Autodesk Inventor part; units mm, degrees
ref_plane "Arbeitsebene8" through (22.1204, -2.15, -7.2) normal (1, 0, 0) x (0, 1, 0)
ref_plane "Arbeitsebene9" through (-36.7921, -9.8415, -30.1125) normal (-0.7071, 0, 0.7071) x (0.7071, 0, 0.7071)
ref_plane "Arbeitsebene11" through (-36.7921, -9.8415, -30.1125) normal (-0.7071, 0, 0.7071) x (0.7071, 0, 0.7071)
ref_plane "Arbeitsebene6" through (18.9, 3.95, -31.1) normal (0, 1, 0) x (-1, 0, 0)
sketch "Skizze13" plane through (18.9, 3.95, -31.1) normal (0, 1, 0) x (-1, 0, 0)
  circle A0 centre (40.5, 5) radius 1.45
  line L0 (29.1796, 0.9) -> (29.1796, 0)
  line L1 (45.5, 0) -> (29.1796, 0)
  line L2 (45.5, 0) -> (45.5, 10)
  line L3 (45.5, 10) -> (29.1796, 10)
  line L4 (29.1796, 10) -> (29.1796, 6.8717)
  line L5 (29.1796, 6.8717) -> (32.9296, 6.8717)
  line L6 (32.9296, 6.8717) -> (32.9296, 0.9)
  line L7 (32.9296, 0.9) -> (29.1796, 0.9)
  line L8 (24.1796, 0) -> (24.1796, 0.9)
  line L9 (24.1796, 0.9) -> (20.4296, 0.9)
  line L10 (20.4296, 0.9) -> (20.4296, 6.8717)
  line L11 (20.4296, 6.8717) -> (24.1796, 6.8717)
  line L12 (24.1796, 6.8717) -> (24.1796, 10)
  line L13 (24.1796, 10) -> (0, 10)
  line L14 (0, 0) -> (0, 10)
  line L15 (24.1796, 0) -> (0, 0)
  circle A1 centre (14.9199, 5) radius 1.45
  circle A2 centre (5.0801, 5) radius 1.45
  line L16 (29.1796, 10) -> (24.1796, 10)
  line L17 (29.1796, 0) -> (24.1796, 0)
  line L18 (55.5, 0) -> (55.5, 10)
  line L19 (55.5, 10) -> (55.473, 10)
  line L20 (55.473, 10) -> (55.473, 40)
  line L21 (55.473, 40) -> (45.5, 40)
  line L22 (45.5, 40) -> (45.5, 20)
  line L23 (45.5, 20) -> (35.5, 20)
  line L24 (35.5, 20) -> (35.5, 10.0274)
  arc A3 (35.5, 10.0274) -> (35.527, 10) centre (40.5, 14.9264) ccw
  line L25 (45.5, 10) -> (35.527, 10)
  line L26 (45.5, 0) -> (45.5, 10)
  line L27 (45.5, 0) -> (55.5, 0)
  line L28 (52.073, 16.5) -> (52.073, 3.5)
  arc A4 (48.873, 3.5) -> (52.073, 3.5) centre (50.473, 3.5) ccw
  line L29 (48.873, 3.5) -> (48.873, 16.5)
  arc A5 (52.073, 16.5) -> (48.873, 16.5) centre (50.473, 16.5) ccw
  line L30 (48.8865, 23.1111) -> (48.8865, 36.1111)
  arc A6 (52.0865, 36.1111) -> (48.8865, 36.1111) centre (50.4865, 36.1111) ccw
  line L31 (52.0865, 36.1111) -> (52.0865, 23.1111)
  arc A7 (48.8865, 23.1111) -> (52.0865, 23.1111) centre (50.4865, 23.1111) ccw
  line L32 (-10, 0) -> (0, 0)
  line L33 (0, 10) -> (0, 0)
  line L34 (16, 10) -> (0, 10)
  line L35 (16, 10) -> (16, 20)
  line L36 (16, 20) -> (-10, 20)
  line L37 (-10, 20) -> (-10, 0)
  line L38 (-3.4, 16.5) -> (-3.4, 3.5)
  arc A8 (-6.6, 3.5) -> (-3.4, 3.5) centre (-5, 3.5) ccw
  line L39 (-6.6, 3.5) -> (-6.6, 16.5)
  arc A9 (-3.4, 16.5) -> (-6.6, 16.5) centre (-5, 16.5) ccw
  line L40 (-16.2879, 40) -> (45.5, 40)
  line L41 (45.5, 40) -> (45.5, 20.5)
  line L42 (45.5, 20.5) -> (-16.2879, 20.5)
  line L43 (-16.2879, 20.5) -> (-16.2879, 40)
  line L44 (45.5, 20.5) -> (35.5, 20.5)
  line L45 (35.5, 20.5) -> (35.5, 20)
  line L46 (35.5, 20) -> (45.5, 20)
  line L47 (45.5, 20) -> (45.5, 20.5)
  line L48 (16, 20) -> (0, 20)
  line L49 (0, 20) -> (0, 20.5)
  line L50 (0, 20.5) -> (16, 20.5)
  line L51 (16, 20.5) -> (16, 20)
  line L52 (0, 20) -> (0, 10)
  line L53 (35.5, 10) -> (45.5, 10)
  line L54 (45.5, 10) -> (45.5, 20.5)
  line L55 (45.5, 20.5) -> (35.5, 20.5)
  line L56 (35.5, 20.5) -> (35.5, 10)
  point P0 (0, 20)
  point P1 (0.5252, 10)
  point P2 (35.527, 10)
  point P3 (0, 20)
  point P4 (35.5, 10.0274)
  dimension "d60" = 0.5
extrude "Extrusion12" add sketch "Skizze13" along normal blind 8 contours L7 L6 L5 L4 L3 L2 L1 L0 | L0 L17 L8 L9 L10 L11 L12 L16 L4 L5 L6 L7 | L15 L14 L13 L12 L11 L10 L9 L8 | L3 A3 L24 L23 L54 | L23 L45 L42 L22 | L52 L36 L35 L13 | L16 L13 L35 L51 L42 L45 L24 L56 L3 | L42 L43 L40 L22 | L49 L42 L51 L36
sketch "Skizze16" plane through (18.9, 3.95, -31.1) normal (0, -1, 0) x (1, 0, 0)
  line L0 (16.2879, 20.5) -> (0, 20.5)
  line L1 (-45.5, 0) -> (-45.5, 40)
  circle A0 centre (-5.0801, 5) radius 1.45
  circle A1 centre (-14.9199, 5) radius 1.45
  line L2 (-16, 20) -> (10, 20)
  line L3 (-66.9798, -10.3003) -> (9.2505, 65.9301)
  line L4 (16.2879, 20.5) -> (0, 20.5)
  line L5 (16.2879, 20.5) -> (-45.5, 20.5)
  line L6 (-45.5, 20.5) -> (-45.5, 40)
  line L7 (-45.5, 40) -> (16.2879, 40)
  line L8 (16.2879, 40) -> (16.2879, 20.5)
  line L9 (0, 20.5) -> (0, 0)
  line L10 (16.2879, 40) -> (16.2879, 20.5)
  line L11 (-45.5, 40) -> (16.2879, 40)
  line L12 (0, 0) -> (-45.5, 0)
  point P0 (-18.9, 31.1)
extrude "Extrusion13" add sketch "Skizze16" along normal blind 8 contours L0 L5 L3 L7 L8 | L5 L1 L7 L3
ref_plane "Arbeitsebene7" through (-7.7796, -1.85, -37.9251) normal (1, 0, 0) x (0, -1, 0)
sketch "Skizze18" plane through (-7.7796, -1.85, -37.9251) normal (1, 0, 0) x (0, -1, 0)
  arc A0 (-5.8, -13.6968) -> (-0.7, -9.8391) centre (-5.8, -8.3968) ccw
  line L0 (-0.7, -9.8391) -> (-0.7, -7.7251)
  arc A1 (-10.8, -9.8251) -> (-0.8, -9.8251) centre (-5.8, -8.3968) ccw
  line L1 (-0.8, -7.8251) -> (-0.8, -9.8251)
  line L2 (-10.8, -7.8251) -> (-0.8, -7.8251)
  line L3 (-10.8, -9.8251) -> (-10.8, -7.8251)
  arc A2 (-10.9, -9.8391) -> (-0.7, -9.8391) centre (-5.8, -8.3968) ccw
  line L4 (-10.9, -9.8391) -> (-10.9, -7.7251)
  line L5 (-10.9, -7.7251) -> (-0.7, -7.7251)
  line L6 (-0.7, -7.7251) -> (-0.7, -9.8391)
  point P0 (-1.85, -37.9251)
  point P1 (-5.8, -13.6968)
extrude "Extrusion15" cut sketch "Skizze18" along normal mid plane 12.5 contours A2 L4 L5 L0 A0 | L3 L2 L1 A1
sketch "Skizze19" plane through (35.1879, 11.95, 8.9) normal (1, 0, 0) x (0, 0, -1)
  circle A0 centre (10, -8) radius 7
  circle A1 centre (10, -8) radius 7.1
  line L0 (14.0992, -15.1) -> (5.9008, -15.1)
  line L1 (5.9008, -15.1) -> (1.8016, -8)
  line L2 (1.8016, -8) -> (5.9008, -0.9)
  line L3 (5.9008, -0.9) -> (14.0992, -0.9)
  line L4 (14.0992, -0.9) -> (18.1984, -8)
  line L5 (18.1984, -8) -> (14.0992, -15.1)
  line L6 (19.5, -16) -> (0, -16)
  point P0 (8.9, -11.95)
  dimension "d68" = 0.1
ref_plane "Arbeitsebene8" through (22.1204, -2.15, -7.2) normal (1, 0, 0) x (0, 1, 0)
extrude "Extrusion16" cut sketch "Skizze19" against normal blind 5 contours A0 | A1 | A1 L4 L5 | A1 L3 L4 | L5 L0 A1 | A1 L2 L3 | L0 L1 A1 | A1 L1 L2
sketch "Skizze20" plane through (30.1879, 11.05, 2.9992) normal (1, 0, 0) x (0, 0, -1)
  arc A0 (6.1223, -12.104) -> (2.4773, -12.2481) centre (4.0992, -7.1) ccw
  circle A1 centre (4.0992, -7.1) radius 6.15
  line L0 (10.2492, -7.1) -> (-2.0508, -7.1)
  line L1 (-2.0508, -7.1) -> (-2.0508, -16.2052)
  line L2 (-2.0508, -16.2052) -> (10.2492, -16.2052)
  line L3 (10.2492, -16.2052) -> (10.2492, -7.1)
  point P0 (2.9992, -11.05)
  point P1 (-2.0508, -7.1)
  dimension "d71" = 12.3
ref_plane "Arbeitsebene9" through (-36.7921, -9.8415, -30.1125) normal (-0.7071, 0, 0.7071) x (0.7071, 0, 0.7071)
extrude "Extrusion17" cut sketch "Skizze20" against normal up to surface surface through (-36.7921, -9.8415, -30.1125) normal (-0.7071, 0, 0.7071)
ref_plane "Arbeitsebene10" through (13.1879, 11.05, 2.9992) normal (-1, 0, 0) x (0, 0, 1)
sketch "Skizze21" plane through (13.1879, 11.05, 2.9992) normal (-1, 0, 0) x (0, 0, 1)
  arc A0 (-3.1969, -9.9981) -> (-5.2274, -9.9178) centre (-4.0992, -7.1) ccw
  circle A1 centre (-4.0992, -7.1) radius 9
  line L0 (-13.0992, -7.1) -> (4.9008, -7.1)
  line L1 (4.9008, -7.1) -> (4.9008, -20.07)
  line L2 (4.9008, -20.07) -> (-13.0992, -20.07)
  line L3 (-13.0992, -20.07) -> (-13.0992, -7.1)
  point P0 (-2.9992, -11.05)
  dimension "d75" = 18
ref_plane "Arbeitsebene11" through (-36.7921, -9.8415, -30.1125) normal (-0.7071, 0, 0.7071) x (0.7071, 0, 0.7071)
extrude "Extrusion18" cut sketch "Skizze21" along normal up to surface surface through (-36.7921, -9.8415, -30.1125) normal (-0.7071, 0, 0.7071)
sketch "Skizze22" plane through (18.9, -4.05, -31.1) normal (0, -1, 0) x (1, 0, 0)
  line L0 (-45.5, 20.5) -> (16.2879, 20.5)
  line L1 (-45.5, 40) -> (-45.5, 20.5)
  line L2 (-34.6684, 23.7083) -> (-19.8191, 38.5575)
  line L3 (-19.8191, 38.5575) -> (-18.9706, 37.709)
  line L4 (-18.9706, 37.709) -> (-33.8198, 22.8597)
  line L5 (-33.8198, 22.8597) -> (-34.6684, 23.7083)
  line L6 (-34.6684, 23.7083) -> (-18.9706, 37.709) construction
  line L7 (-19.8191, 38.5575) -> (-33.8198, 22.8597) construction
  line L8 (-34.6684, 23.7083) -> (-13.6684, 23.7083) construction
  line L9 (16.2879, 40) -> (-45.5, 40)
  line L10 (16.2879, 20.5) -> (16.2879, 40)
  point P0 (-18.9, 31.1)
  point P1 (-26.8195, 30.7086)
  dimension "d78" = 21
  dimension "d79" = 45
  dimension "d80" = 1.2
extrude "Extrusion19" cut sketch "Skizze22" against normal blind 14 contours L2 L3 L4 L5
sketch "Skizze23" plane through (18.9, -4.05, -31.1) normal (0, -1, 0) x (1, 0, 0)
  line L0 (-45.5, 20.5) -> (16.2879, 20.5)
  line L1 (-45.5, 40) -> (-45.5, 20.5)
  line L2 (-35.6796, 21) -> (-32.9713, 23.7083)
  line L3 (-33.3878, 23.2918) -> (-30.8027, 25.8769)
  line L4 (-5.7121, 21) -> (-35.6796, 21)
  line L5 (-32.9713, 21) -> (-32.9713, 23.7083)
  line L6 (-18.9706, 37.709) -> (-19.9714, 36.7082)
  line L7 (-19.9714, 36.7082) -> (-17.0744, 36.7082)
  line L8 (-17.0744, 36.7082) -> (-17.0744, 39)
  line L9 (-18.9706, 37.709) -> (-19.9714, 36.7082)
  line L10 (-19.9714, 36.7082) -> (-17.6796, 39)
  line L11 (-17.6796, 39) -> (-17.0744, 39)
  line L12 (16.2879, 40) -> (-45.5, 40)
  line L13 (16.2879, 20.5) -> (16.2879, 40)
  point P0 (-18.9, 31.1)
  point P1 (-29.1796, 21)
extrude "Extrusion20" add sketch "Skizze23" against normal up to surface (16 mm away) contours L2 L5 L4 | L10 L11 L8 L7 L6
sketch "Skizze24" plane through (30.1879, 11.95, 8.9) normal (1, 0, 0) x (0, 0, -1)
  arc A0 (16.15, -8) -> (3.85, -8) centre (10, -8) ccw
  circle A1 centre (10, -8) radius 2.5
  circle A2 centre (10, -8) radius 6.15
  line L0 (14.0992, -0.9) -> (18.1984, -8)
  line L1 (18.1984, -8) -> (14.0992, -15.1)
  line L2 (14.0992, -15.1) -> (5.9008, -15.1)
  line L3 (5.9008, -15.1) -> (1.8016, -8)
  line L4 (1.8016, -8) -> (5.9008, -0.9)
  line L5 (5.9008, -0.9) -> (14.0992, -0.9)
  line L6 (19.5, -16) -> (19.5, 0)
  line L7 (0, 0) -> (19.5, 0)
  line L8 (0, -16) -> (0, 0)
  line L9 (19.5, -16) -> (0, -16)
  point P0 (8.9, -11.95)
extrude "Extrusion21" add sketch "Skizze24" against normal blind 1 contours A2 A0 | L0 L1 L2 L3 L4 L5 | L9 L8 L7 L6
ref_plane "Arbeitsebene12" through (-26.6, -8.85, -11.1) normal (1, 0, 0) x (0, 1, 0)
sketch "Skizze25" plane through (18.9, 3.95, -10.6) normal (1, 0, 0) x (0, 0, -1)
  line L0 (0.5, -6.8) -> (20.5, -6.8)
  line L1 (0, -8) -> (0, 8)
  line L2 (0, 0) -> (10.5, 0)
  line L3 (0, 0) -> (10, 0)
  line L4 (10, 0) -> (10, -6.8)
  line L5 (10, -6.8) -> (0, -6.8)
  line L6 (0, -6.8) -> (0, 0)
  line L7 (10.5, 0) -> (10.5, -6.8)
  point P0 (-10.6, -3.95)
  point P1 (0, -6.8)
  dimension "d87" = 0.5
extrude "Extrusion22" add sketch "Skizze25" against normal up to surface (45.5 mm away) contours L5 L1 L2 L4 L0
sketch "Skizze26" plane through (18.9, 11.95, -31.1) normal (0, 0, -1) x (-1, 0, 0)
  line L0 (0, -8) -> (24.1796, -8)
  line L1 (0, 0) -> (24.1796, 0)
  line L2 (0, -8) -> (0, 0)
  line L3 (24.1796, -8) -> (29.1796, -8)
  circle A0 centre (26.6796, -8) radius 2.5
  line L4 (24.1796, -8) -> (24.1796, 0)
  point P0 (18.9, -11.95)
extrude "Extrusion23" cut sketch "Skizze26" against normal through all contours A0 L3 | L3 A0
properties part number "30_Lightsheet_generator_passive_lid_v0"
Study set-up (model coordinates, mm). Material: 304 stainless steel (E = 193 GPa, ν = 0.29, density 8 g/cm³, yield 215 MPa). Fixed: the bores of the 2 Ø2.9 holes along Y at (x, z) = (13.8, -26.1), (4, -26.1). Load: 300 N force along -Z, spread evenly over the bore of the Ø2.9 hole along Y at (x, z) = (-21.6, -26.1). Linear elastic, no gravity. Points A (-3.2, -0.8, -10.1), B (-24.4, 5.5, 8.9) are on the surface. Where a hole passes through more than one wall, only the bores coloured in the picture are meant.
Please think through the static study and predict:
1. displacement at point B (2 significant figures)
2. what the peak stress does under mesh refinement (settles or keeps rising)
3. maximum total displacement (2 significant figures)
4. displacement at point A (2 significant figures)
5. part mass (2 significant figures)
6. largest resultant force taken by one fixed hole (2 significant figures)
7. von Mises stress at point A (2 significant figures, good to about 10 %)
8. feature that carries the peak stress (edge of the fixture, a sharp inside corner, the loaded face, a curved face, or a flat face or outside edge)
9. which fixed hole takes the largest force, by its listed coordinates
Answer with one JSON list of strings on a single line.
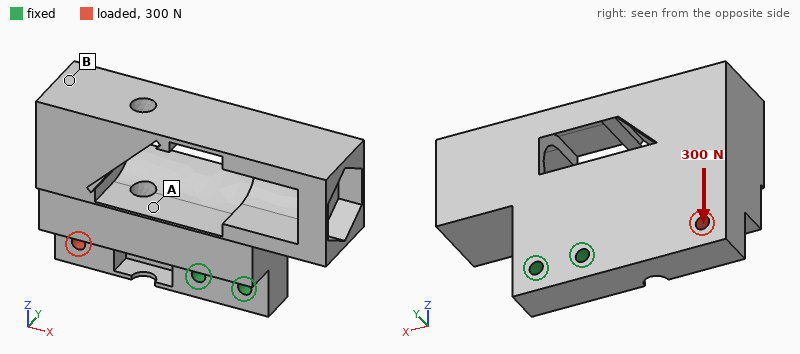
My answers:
["6.6 µm", "keeps rising", "6.9 µm", "2.0 µm", "160 g", "900 N", "4.8 MPa", "edge of the fixture", "(4, -26.1)"]
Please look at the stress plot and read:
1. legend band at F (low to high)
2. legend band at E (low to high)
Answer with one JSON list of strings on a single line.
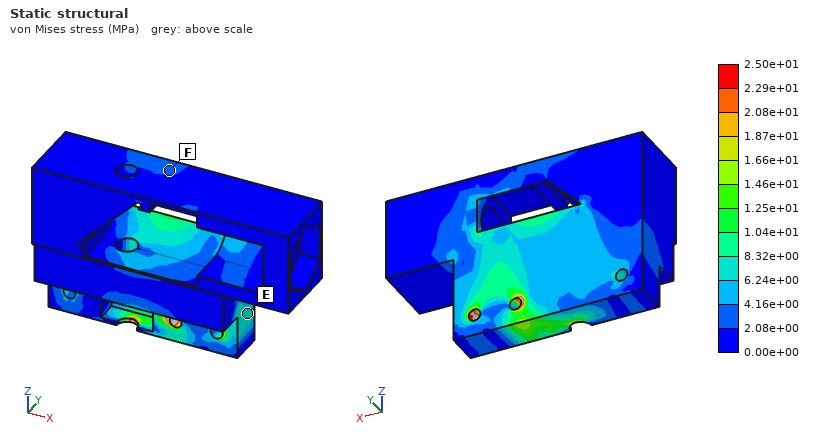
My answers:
["2.08e+00 to 4.16e+00 MPa", "6.24e+00 to 8.32e+00 MPa"]
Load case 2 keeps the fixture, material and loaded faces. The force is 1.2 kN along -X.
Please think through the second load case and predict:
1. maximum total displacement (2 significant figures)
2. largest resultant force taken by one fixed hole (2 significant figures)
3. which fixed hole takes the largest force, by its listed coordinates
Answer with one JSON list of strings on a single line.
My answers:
["4.6 µm", "970 N", "(4, -26.1)"]
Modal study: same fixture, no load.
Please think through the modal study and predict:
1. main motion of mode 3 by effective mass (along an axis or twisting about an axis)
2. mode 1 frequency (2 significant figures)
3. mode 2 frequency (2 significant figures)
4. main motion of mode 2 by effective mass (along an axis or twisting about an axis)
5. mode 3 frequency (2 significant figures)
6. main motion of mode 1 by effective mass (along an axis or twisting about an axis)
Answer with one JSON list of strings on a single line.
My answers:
["twisting about Z", "2500 Hz", "3700 Hz", "along X", "3800 Hz", "along Y"]
